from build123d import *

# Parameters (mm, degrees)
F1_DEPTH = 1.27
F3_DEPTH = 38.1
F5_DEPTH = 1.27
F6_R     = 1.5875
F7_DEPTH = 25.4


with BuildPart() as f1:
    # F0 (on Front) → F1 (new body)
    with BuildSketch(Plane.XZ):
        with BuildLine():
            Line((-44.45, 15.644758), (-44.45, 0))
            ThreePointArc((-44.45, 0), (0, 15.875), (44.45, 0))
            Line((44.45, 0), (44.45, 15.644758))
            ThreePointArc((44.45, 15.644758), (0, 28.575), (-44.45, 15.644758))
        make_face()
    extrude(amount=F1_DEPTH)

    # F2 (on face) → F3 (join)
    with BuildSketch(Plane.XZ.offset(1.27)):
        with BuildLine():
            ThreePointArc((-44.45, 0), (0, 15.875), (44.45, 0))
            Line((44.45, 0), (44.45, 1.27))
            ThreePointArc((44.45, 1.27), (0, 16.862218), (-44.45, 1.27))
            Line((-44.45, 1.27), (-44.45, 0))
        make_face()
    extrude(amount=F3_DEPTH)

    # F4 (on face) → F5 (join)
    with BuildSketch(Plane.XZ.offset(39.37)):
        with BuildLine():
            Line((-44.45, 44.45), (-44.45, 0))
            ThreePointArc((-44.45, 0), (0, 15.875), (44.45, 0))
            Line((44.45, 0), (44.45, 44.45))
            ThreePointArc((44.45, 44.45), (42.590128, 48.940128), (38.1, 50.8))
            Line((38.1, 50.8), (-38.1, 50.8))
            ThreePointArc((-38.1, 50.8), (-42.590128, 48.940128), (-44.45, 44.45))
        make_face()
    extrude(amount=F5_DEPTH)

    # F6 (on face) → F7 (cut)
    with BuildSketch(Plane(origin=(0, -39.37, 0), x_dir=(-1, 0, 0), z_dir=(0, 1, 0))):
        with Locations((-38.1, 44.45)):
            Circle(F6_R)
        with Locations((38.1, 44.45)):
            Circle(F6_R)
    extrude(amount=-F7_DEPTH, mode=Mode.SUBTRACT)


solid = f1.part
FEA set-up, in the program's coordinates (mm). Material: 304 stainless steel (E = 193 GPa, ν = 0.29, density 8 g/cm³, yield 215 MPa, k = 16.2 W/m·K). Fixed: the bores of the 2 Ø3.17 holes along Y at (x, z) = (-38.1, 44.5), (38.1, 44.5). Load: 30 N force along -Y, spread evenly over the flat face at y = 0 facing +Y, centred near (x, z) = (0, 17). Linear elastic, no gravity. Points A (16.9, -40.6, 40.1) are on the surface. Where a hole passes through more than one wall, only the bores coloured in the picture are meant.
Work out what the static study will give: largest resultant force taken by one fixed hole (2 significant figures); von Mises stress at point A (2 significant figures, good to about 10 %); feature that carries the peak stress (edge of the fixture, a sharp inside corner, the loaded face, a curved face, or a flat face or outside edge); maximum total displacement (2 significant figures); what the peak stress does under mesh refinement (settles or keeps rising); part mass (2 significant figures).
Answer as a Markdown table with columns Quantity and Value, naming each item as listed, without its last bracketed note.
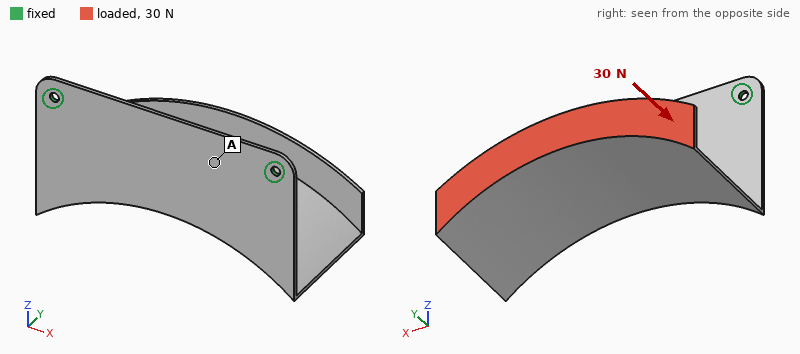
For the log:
| Quantity | Value |
|---|---|
| largest resultant force taken by one fixed hole | 16 N |
| von Mises stress at point A | 15 MPa |
| feature that carries the peak stress | edge of the fixture |
| maximum total displacement | 0.32 mm |
| what the peak stress does under mesh refinement | keeps rising |
| part mass | 77 g |
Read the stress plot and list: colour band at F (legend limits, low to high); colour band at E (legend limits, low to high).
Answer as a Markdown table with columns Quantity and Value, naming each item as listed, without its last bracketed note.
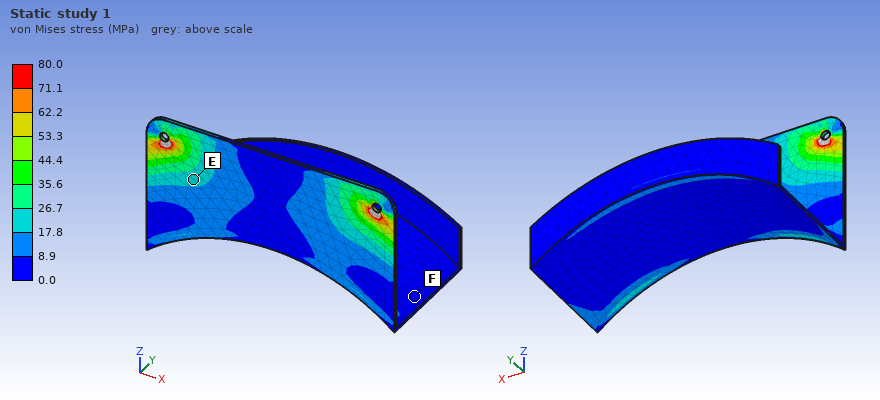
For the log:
| Quantity | Value |
|---|---|
| colour band at F | 0.0 to 8.9 MPa |
| colour band at E | 17.8 to 26.7 MPa |
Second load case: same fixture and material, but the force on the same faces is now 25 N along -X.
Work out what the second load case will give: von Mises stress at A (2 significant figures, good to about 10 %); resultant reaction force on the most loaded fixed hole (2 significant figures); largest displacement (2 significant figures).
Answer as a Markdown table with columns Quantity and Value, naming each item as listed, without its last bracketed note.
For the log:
| Quantity | Value |
|---|---|
| von Mises stress at A | 10.0 MPa |
| resultant reaction force on the most loaded fixed hole | 21 N |
| largest displacement | 0.19 mm |
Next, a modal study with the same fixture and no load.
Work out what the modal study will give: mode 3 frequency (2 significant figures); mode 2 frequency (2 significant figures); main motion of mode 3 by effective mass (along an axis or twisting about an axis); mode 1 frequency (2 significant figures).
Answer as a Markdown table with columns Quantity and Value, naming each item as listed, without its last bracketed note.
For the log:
| Quantity | Value |
|---|---|
| mode 3 frequency | 510 Hz |
| mode 2 frequency | 320 Hz |
| main motion of mode 3 by effective mass | along Y |
| mode 1 frequency | 180 Hz |
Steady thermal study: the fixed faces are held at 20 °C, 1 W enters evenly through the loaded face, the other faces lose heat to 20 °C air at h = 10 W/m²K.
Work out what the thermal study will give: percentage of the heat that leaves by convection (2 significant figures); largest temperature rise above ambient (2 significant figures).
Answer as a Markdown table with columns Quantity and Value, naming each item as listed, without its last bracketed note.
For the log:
| Quantity | Value |
|---|---|
| percentage of the heat that leaves by convection | 92 % |
| largest temperature rise above ambient | 17 K |
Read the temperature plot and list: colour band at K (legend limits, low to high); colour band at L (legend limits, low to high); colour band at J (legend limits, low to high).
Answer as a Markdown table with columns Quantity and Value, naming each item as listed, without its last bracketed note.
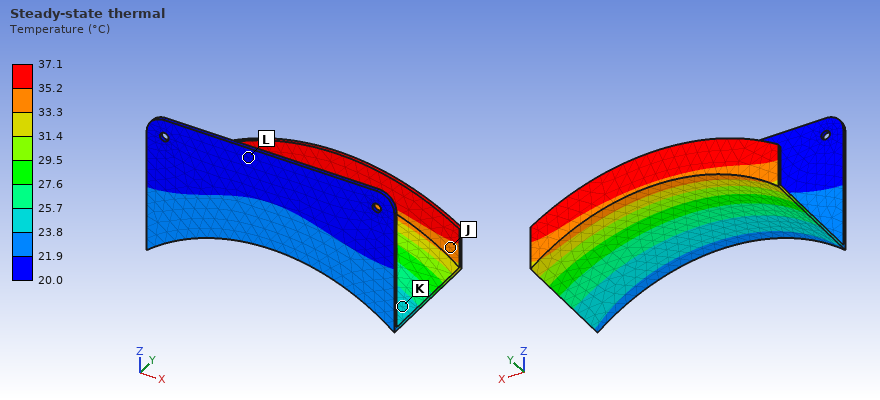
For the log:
| Quantity | Value |
|---|---|
| colour band at K | 23.8 to 25.7 °C |
| colour band at L | 20.0 to 21.9 °C |
| colour band at J | 33.3 to 35.2 °C |
